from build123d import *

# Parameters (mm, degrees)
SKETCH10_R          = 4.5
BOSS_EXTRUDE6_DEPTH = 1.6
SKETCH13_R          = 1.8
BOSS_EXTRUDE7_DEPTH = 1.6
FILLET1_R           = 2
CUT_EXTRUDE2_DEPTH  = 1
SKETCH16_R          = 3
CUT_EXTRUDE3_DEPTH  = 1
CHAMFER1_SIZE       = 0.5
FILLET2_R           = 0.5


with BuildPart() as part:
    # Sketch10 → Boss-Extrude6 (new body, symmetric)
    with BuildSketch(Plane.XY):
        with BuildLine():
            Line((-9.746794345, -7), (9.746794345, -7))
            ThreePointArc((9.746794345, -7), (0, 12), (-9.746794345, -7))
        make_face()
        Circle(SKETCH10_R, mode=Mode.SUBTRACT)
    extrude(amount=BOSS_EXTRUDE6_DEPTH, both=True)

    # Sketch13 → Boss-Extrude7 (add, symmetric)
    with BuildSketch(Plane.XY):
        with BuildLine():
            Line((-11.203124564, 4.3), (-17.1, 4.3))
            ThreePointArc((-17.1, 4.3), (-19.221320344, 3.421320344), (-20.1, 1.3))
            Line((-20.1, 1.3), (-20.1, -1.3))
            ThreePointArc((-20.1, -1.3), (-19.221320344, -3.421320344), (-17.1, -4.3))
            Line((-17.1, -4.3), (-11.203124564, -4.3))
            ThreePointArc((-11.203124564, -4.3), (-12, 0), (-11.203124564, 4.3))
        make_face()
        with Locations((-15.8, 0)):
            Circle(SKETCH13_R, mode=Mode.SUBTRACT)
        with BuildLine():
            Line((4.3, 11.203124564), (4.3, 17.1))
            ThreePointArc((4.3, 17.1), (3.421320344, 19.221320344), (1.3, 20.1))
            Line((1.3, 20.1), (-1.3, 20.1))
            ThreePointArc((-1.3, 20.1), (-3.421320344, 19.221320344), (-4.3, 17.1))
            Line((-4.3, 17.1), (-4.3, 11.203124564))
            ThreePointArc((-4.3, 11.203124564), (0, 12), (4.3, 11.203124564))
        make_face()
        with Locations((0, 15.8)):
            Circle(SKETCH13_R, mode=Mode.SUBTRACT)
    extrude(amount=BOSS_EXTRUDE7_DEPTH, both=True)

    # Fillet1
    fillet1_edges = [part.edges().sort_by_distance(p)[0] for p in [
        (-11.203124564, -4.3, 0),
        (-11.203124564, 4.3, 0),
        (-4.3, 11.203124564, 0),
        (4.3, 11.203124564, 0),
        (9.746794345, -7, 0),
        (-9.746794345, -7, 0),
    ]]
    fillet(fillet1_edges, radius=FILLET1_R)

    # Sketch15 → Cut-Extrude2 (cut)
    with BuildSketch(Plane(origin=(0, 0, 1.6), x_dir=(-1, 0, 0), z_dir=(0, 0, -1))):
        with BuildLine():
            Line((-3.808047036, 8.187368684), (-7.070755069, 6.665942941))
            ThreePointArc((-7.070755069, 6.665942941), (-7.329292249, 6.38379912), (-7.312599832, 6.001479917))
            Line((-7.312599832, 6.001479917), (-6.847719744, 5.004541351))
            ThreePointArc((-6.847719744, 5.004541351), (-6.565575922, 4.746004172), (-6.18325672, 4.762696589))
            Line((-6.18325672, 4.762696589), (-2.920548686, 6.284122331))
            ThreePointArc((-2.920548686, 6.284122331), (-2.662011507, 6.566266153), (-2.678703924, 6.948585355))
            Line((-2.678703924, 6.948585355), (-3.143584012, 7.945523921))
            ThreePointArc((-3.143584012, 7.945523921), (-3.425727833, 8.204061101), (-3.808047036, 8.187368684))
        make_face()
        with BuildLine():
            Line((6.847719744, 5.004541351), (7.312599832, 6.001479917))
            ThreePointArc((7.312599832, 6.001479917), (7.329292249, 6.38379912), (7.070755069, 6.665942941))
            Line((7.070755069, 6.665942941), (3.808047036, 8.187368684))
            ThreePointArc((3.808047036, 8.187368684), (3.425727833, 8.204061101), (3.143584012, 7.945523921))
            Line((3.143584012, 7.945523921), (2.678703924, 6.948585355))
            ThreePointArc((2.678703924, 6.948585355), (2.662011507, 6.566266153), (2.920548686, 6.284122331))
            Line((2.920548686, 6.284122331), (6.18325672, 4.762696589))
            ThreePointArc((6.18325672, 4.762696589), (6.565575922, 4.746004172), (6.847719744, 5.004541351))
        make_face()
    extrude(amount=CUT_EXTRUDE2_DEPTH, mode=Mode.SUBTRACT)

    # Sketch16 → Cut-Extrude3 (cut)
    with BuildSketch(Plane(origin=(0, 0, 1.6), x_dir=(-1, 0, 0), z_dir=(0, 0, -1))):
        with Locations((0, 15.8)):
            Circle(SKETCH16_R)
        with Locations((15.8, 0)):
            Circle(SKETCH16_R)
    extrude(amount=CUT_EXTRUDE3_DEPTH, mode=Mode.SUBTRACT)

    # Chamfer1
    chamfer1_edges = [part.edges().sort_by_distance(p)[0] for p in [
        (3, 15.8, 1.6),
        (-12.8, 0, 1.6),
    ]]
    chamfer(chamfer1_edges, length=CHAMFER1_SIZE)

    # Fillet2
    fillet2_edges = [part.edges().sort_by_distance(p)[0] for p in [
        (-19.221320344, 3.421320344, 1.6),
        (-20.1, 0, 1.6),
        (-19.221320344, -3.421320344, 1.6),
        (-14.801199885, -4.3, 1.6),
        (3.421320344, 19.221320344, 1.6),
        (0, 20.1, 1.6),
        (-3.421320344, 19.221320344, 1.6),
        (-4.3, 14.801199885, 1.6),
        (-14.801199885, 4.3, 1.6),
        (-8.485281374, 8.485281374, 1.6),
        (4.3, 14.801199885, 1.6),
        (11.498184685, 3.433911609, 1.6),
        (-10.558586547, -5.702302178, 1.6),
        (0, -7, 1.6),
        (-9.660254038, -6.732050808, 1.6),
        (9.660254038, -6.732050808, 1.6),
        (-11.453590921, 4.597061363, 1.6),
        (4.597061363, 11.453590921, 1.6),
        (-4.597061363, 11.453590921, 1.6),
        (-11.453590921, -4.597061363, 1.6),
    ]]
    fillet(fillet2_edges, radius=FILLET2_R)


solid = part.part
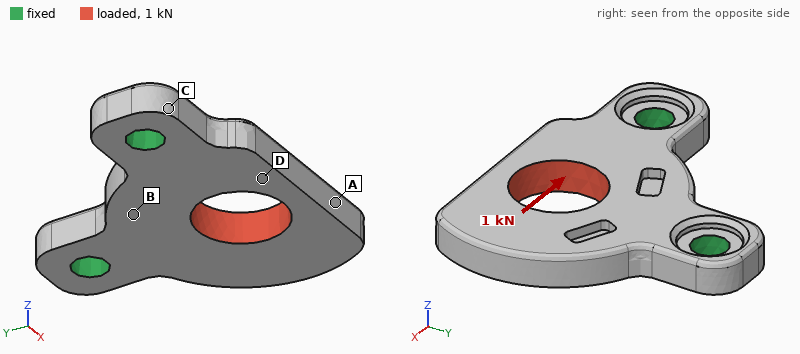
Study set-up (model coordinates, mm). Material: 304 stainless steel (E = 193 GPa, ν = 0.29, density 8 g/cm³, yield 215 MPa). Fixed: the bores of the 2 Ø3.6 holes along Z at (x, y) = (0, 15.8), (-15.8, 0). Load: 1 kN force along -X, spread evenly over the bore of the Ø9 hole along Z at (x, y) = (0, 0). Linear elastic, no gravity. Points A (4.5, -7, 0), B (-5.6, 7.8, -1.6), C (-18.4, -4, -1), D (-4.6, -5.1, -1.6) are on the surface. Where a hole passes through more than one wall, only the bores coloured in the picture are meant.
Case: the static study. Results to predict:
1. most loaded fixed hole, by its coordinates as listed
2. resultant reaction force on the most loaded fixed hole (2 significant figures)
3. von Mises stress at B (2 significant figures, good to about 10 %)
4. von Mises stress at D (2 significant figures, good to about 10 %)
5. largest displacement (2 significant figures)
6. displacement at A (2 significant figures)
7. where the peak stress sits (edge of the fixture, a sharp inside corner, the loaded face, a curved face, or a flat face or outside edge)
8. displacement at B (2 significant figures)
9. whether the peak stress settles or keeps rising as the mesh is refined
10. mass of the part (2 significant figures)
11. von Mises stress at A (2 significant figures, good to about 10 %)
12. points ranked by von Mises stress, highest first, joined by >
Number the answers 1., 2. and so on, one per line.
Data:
1. (-15.8, 0)
2. 840 N
3. 14 MPa
4. 37 MPa
5. 6.0 µm
6. 5.4 µm
7. edge of the fixture
8. 1.4 µm
9. keeps rising
10. 11 g
11. 25 MPa
12. D > A > B > C
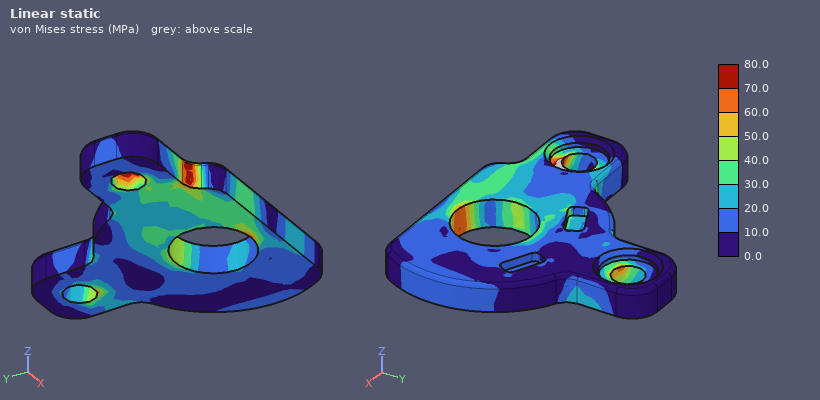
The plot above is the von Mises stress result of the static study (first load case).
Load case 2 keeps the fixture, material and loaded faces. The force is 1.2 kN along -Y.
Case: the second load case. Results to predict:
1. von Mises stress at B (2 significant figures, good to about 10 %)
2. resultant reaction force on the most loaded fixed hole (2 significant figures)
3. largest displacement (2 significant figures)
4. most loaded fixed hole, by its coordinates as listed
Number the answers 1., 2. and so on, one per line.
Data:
1. 25 MPa
2. 1.0 kN
3. 7.6 µm
4. (0, 15.8)
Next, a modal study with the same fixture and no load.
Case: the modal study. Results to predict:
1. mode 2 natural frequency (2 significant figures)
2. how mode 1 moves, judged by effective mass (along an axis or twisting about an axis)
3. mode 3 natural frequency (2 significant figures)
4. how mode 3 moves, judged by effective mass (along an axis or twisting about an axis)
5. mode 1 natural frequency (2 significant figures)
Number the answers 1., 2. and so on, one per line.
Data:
1. 17 kHz
2. along Z
3. 24 kHz
4. along Z
5. 5300 Hz
